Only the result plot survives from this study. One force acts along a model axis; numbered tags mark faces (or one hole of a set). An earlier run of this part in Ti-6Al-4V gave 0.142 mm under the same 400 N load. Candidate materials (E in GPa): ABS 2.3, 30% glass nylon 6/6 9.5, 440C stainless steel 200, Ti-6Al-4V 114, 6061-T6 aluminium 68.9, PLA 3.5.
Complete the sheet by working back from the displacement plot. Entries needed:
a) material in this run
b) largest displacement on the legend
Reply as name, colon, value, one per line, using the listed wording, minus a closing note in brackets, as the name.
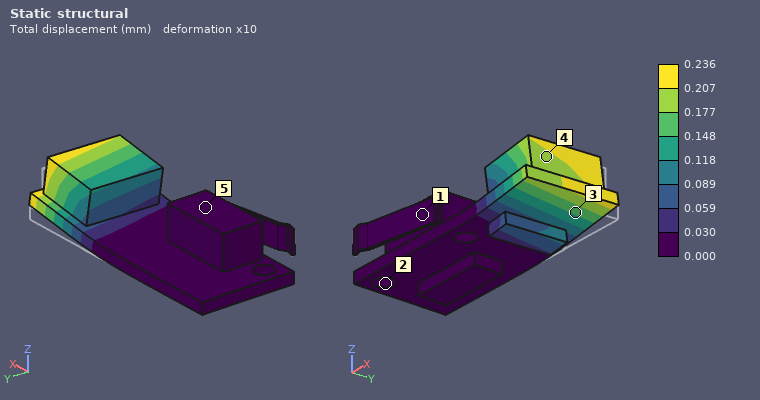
material in this run: 6061-T6 aluminium
largest displacement on the legend: 0.236 mm
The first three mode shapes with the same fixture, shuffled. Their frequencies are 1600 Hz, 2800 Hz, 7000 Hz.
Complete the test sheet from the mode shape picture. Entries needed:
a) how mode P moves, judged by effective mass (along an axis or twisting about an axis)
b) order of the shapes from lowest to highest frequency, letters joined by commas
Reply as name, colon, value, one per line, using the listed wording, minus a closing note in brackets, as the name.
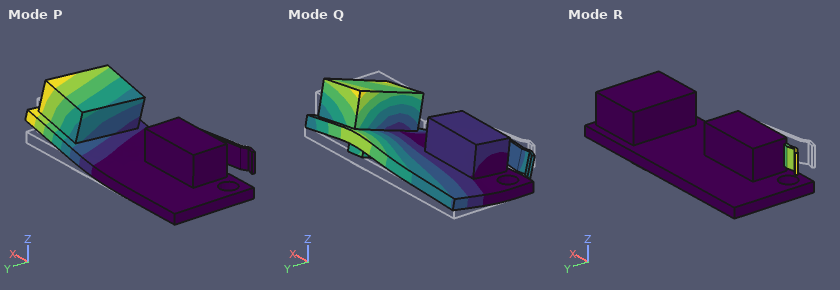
how mode P moves, judged by effective mass: along Z
order of the shapes from lowest to highest frequency, letters joined by commas: R, P, Q
